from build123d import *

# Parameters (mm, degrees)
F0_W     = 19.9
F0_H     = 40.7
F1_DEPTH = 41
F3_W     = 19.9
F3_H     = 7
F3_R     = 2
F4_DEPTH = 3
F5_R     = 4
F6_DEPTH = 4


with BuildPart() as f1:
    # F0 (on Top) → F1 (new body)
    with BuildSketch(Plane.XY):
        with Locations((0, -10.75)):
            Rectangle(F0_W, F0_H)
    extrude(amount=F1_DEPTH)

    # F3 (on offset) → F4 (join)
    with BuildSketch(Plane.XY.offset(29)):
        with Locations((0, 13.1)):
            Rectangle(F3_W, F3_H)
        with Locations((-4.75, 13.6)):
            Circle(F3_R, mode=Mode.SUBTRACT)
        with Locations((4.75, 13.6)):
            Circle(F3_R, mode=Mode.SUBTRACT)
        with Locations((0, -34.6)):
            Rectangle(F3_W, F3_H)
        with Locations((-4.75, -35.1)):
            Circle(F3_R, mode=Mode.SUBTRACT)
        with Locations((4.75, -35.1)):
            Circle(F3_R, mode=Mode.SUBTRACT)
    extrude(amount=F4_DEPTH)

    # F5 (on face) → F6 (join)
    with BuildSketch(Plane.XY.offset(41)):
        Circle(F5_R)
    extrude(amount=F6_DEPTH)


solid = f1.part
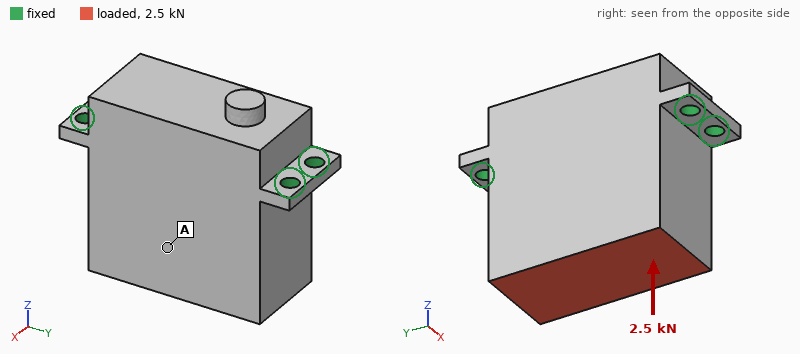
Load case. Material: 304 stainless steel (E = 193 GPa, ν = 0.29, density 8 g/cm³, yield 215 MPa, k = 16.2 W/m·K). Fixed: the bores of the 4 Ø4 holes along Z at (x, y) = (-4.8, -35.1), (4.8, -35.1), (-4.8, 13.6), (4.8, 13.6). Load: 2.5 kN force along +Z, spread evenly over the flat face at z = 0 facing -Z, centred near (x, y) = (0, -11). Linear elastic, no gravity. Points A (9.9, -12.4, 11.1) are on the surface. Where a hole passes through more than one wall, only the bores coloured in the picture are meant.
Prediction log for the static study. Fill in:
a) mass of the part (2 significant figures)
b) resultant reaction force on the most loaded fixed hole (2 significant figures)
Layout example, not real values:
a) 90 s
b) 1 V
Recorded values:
a) 270 g
b) 630 N
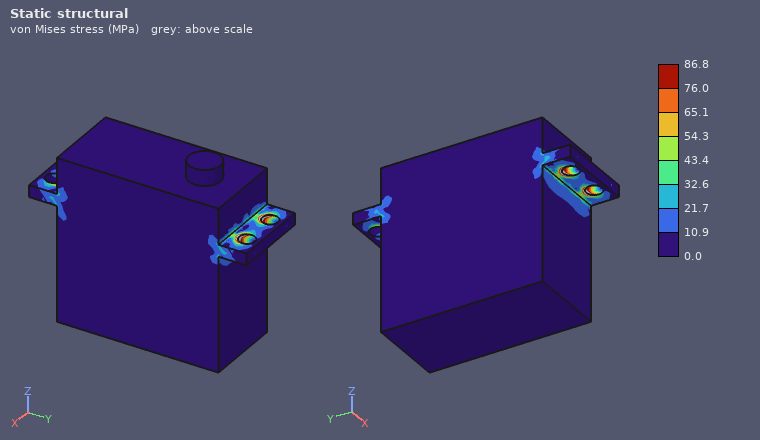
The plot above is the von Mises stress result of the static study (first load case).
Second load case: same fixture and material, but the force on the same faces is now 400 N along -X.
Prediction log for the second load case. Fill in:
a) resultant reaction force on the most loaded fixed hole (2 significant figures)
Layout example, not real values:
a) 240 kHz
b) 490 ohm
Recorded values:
a) 500 N
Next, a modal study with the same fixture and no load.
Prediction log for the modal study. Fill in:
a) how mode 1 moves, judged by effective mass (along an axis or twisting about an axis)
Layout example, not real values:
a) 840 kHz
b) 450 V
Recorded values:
a) along X
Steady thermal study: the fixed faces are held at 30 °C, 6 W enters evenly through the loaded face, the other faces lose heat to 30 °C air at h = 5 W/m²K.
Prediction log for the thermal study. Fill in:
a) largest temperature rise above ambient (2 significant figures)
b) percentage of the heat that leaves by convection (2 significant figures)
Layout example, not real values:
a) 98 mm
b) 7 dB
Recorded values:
a) 28 K
b) 9.1 %
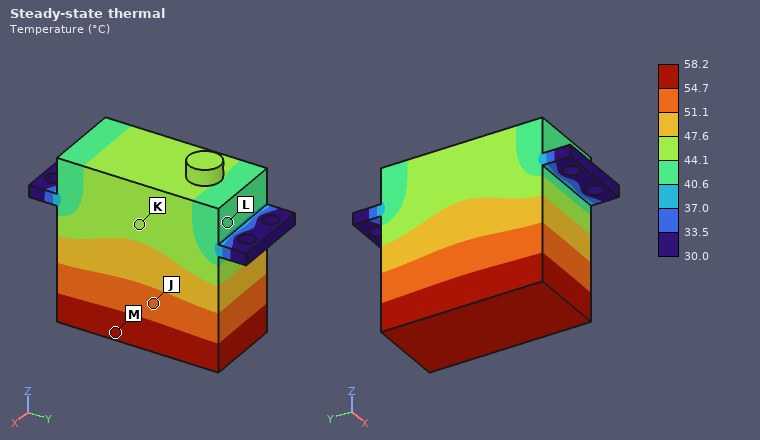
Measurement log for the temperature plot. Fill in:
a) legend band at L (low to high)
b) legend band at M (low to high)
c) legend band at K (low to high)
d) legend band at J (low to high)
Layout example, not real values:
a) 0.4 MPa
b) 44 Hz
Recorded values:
a) 40.6 to 44.1 °C
b) 54.7 to 58.2 °C
c) 44.1 to 47.6 °C
d) 51.1 to 54.7 °C
